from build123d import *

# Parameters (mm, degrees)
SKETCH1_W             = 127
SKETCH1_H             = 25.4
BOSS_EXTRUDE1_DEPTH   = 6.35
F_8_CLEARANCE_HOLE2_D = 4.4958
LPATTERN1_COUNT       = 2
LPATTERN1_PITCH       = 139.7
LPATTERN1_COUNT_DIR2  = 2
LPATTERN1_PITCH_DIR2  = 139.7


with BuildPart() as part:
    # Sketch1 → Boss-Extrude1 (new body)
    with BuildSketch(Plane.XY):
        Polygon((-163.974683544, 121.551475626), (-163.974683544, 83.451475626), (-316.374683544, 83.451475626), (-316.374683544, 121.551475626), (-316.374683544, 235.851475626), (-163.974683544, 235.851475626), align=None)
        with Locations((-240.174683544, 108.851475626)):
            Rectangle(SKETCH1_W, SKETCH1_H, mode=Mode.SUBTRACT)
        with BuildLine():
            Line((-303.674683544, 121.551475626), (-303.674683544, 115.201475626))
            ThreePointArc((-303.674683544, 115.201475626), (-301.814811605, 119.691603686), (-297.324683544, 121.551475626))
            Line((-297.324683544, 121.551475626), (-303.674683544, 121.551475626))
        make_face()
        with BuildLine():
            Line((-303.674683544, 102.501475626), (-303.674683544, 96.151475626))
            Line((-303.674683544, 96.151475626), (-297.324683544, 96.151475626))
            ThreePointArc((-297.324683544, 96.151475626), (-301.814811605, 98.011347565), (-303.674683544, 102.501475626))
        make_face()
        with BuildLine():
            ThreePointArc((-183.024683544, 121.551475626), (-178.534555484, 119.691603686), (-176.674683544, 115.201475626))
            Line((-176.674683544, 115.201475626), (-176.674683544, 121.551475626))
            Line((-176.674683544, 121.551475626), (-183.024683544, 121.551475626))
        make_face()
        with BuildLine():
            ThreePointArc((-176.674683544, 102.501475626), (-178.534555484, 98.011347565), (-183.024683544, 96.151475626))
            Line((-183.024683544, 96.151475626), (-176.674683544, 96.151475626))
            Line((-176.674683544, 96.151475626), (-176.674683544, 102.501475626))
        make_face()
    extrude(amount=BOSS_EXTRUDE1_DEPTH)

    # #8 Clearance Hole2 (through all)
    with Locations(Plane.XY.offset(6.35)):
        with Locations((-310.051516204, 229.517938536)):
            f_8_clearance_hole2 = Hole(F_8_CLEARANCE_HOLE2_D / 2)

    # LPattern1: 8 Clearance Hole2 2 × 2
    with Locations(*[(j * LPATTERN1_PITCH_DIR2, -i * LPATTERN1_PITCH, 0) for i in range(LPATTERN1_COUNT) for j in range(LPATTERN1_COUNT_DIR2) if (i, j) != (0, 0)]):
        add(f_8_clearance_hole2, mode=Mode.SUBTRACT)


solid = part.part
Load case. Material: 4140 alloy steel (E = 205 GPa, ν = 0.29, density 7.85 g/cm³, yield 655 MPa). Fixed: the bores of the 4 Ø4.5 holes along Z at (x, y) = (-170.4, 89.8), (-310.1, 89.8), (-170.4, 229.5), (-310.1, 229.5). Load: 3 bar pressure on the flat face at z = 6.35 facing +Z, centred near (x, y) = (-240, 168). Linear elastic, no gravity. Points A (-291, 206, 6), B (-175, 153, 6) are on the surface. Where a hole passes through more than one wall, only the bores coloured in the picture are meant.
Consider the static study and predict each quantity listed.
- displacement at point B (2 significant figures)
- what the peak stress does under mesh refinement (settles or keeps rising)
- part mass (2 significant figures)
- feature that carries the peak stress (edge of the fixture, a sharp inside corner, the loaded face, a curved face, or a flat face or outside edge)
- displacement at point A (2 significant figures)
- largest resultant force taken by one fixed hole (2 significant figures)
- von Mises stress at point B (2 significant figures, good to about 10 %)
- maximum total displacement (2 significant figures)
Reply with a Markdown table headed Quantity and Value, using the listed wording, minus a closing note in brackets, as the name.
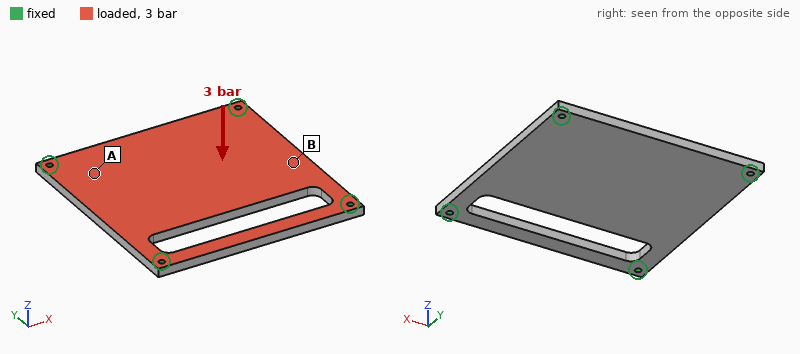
| Quantity | Value |
|---|---|
| displacement at point B | 0.17 mm |
| what the peak stress does under mesh refinement | keeps rising |
| part mass | 1000 g |
| feature that carries the peak stress | edge of the fixture |
| displacement at point A | 0.10 mm |
| largest resultant force taken by one fixed hole | 1.7 kN |
| von Mises stress at point B | 63 MPa |
| maximum total displacement | 0.33 mm |
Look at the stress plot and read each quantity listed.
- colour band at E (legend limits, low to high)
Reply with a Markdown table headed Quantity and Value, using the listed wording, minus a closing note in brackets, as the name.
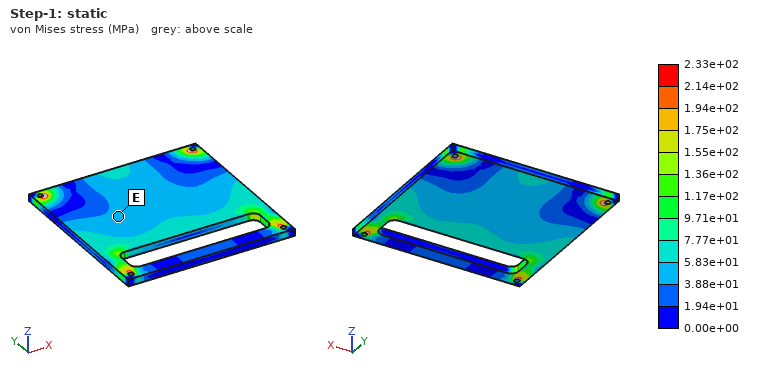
| Quantity | Value |
|---|---|
| colour band at E | 3.88e+01 to 5.83e+01 MPa |
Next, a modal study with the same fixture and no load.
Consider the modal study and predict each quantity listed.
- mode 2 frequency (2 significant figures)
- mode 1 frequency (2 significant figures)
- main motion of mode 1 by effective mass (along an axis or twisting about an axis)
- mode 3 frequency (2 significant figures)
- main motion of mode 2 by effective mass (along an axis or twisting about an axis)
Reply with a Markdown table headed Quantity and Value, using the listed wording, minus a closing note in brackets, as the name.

| Quantity | Value |
|---|---|
| mode 2 frequency | 1600 Hz |
| mode 1 frequency | 840 Hz |
| main motion of mode 1 by effective mass | along Z |
| mode 3 frequency | 1800 Hz |
| main motion of mode 2 by effective mass | twisting about Y |
